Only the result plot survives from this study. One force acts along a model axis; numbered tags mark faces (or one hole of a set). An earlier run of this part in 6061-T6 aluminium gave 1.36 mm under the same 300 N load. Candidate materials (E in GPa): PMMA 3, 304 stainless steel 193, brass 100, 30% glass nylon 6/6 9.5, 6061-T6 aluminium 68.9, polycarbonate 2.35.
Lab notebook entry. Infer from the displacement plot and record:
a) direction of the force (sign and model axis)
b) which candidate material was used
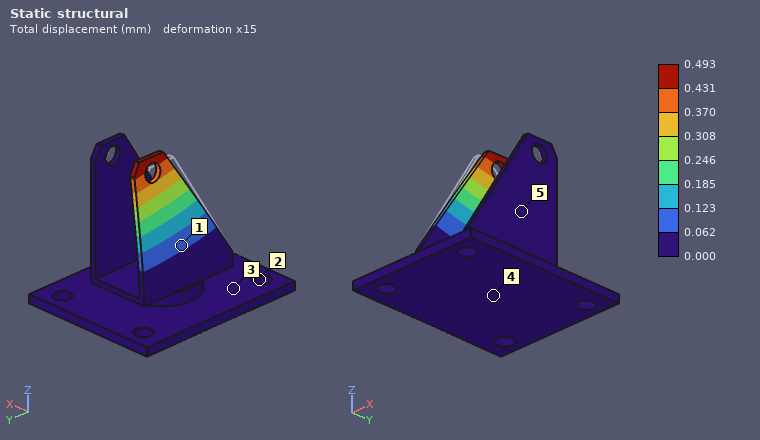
+X
304 stainless steel
